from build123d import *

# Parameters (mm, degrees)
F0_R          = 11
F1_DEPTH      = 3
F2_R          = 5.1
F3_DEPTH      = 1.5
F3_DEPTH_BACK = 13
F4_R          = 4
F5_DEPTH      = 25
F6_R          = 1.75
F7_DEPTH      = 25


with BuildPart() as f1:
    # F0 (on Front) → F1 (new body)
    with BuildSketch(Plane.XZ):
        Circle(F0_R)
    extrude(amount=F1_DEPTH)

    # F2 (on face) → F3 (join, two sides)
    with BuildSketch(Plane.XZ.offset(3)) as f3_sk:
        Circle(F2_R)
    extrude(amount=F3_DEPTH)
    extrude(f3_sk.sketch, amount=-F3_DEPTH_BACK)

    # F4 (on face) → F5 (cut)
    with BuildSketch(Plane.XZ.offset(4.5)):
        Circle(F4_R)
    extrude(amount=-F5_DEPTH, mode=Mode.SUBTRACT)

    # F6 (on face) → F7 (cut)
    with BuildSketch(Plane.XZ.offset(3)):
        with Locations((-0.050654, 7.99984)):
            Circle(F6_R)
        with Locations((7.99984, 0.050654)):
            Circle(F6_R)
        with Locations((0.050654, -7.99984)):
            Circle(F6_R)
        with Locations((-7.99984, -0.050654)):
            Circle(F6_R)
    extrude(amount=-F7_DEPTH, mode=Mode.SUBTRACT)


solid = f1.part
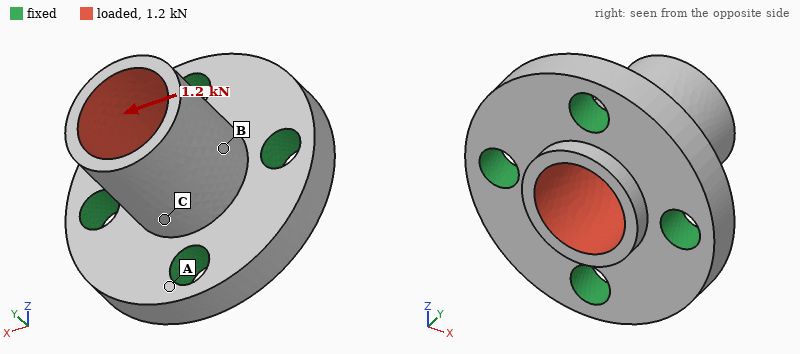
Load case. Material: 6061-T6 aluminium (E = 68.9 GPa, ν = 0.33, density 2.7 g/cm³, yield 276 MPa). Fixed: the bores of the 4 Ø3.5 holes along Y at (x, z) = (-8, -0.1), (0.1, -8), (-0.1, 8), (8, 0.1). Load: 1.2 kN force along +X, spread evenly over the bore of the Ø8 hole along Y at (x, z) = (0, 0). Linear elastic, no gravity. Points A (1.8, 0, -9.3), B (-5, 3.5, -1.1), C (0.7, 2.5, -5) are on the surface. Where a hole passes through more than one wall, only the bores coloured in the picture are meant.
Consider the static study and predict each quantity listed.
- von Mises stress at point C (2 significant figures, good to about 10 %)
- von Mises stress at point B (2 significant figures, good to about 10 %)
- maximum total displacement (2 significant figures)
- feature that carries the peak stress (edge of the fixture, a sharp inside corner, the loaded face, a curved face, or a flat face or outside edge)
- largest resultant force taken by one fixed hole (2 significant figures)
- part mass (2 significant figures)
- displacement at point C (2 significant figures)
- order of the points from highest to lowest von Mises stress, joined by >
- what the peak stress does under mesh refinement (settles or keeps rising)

51 MPa
22 MPa
22 µm
a sharp inside corner
510 N
3.3 g
7.1 µm
C > B > A
keeps rising
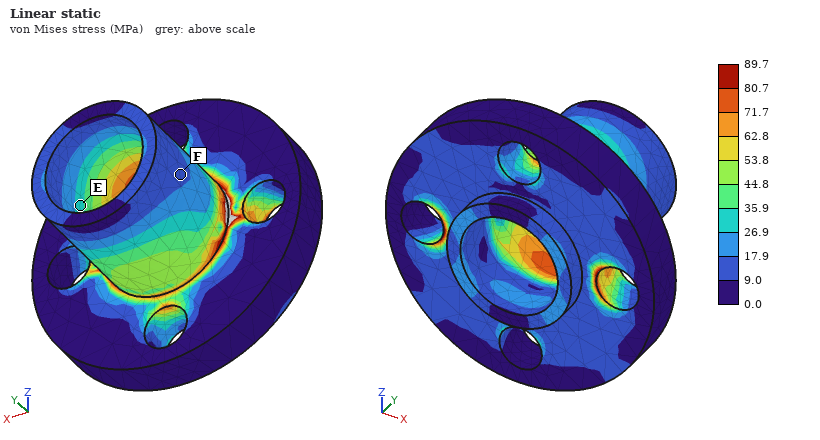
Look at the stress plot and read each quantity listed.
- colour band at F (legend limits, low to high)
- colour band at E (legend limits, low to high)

9.0 to 17.9 MPa
26.9 to 35.9 MPa
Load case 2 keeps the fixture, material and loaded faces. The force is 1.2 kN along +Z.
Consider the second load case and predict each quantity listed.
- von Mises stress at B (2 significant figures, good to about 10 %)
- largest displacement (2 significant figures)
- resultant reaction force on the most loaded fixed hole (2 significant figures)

49 MPa
22 µm
510 N
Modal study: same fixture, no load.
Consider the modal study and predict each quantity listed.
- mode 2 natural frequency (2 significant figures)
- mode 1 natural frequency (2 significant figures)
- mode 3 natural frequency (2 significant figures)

39 kHz
39 kHz
42 kHz
